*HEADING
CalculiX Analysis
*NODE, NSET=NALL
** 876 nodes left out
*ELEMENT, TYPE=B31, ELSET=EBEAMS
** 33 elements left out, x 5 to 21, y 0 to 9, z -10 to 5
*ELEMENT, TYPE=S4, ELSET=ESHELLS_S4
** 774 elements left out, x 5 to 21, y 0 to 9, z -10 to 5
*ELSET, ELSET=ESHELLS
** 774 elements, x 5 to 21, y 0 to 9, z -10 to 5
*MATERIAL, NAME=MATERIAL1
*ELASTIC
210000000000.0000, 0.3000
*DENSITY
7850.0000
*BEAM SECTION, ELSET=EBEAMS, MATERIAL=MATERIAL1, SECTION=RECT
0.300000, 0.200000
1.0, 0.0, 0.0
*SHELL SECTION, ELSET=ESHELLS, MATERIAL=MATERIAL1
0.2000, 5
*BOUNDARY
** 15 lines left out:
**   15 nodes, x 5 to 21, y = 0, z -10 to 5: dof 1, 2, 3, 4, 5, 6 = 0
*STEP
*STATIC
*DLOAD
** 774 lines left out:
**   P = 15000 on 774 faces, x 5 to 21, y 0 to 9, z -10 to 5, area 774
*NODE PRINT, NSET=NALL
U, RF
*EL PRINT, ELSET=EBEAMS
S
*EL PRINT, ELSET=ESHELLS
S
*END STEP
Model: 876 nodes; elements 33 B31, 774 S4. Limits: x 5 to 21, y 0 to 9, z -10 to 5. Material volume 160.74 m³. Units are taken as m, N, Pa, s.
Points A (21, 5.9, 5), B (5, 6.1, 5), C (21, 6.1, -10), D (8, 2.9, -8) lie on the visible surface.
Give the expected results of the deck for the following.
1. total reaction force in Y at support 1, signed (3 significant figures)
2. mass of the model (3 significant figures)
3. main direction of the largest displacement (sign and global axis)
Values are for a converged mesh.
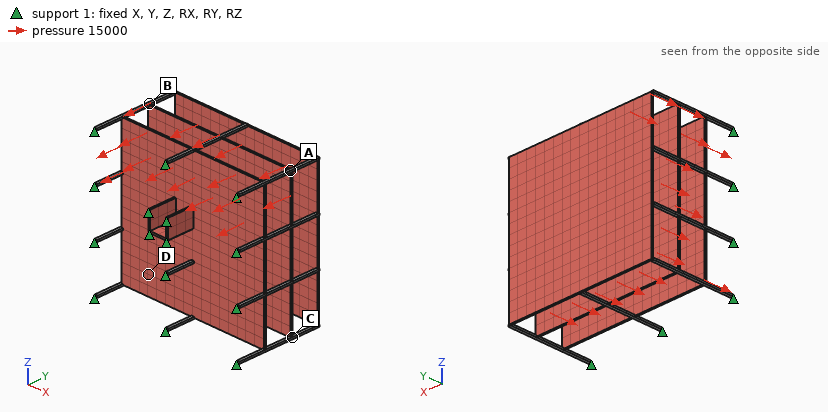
1.08e+07 N
1.26e+06 kg
-Y
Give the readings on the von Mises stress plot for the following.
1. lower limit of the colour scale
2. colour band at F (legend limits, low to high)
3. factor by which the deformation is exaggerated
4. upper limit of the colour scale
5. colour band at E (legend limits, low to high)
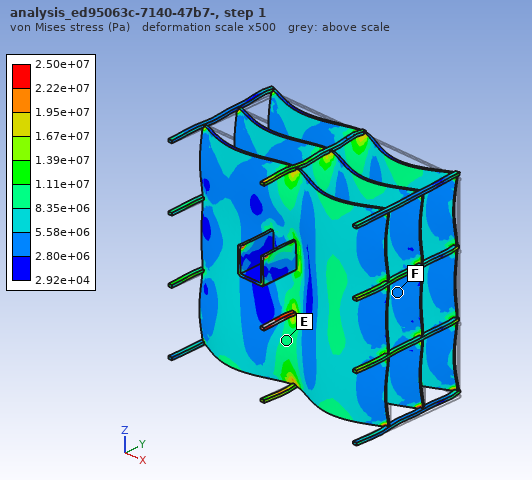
2.92e+04 Pa
2.80e+06 to 5.58e+06 Pa
500
2.50e+07 Pa
8.35e+06 to 1.11e+07 Pa
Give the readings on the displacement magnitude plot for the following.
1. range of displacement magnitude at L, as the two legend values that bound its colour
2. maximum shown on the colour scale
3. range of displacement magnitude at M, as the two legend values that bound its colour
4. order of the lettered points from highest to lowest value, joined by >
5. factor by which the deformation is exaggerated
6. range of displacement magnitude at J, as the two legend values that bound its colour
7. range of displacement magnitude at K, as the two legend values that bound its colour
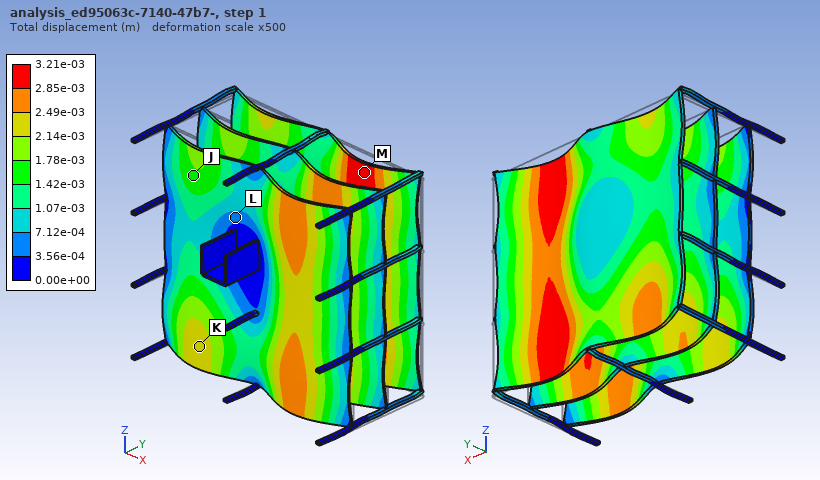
3.56e-04 to 7.12e-04 m
3.21e-03 m
2.85e-03 to 3.21e-03 m
M > K > J > L
500
1.42e-03 to 1.78e-03 m
2.14e-03 to 2.49e-03 m
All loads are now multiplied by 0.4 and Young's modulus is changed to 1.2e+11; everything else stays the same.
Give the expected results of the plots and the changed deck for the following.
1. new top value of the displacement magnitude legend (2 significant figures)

0.0022 m
